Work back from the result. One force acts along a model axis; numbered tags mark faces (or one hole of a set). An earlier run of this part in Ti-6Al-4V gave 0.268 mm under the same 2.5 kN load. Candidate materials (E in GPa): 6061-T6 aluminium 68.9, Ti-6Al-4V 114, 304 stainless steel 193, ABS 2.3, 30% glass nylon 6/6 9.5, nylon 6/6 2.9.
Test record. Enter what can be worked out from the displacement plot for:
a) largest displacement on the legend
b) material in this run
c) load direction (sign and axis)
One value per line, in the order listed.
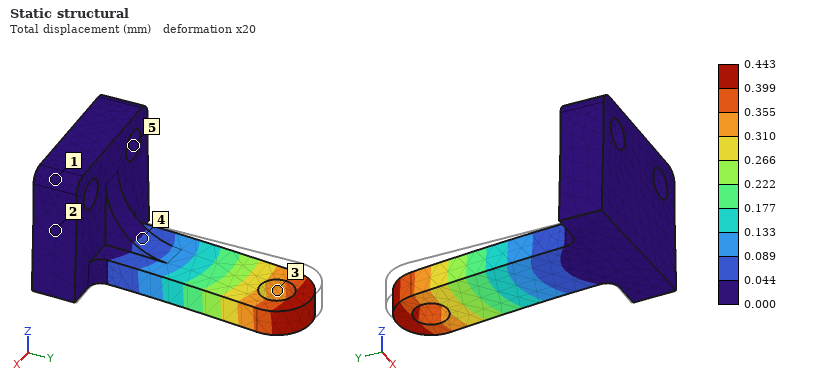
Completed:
0.443 mm
6061-T6 aluminium
+X
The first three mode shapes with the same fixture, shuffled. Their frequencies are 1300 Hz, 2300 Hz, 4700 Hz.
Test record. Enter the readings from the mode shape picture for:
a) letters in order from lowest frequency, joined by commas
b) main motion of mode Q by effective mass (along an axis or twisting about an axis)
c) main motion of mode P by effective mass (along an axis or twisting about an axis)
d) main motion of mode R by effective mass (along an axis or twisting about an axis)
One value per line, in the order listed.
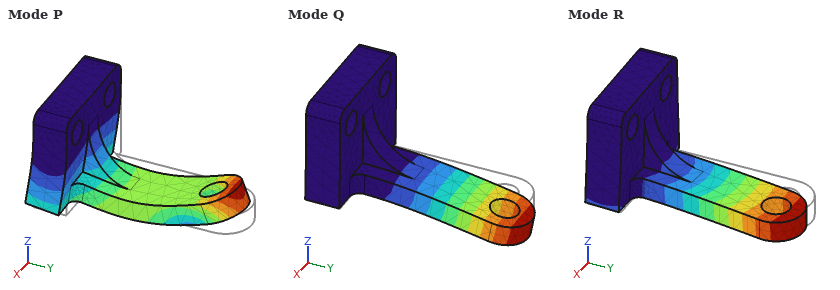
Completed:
Q, R, P
along Z
along Y
along X
